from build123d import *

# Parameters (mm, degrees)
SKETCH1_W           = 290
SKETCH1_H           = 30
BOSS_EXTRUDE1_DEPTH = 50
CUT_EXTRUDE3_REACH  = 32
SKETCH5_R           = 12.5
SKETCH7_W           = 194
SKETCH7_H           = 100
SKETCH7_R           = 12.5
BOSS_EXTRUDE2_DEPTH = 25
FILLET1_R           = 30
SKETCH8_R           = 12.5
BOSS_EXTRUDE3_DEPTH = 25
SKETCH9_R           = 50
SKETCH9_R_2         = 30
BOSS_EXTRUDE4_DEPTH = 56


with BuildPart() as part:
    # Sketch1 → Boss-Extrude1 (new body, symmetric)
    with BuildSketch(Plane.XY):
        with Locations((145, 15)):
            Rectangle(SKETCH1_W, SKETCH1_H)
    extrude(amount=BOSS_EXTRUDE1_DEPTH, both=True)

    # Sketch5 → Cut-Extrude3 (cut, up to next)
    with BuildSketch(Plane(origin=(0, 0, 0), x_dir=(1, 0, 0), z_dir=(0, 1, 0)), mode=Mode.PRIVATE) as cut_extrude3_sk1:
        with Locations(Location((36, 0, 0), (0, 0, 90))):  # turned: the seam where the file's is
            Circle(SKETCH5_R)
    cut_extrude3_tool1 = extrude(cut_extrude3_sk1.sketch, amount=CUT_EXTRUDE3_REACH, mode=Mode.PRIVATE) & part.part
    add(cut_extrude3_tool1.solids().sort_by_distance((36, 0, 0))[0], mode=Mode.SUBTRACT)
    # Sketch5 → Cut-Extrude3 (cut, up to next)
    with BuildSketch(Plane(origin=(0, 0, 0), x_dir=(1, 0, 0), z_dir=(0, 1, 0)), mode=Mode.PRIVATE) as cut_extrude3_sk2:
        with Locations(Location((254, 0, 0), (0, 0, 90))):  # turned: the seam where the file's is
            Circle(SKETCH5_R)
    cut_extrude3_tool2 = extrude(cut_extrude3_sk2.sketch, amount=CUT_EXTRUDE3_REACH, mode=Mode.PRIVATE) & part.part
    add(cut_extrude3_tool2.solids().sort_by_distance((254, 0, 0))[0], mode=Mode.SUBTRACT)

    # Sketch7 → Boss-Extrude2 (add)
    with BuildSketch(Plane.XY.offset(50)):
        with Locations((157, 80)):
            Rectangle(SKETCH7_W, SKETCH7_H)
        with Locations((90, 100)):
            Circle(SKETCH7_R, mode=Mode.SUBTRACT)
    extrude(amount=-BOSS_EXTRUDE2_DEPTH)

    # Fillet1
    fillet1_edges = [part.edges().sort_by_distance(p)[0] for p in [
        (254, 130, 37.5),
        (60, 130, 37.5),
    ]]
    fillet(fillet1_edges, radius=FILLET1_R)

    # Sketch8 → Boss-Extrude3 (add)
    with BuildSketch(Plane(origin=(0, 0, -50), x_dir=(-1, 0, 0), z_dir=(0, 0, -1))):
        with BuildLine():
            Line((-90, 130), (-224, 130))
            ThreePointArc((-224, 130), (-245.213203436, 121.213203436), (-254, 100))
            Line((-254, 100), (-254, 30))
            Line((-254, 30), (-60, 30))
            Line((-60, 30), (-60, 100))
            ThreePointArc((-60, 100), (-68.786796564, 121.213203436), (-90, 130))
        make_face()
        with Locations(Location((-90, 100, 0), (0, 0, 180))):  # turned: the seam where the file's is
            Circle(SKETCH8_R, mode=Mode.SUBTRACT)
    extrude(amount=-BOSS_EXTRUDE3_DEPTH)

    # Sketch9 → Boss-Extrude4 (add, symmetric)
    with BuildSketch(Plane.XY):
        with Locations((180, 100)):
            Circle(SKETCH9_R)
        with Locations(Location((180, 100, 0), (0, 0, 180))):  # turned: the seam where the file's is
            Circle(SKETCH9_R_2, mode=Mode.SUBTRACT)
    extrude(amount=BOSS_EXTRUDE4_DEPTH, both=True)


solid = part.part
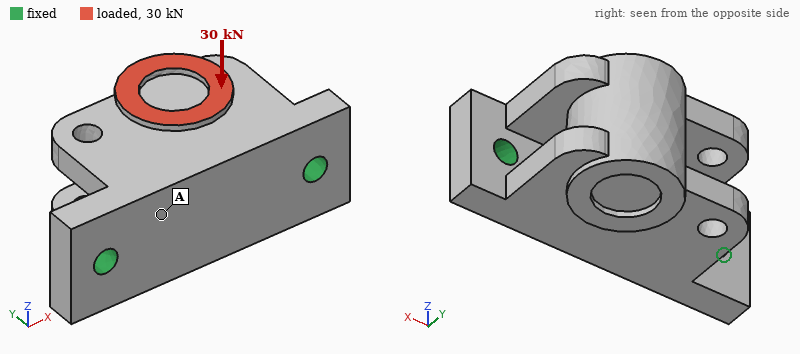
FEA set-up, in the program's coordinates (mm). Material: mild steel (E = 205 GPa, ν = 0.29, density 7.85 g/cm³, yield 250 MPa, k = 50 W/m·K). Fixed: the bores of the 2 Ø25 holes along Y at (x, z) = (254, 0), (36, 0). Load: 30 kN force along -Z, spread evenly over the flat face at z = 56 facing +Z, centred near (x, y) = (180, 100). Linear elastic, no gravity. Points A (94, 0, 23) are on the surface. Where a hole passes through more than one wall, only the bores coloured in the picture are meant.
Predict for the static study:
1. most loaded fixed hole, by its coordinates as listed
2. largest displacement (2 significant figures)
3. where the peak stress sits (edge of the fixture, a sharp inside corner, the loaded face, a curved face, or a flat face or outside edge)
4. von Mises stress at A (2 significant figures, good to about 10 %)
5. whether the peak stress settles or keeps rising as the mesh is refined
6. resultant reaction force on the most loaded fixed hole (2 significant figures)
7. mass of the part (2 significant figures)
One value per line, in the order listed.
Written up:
(254, 0)
0.11 mm
edge of the fixture
13 MPa
keeps rising
20 kN
17 kg
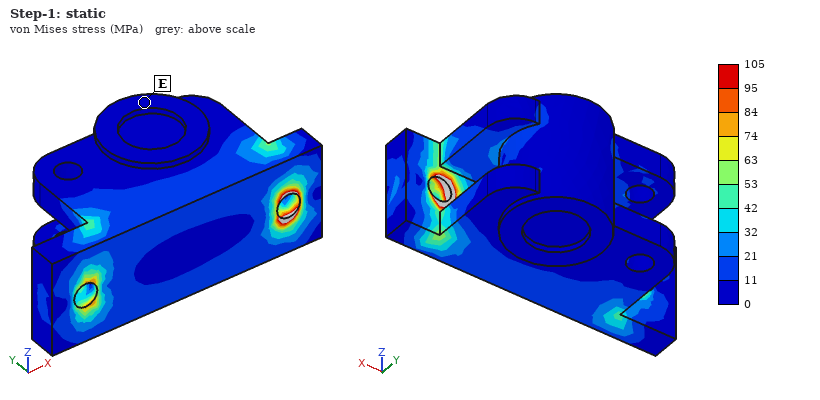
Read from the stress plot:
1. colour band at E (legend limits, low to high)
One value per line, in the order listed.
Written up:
0 to 11 MPa
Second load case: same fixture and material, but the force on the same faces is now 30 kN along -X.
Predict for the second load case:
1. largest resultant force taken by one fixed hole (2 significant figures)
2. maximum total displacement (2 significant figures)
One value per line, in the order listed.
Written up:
21 kN
21 µm
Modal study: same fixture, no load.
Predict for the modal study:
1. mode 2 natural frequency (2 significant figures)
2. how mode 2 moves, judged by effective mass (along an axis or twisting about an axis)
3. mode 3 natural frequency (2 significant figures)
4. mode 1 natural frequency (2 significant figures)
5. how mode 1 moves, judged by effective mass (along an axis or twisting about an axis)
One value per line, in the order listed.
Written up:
2700 Hz
along Y
3200 Hz
1100 Hz
along Z
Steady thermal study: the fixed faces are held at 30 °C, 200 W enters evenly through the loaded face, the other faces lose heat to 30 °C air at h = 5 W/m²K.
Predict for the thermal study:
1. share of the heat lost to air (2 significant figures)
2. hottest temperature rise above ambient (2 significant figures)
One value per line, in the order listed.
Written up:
15 %
81 K
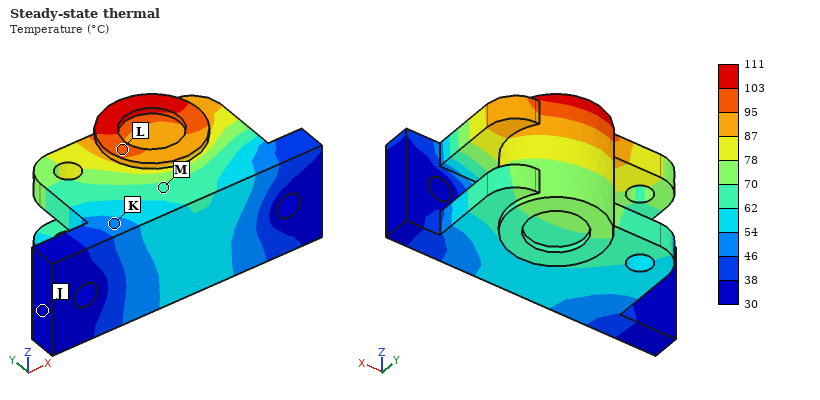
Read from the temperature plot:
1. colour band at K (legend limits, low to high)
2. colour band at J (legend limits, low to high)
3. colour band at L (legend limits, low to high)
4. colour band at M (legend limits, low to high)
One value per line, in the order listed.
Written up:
46 to 54 °C
30 to 38 °C
95 to 103 °C
62 to 70 °C
